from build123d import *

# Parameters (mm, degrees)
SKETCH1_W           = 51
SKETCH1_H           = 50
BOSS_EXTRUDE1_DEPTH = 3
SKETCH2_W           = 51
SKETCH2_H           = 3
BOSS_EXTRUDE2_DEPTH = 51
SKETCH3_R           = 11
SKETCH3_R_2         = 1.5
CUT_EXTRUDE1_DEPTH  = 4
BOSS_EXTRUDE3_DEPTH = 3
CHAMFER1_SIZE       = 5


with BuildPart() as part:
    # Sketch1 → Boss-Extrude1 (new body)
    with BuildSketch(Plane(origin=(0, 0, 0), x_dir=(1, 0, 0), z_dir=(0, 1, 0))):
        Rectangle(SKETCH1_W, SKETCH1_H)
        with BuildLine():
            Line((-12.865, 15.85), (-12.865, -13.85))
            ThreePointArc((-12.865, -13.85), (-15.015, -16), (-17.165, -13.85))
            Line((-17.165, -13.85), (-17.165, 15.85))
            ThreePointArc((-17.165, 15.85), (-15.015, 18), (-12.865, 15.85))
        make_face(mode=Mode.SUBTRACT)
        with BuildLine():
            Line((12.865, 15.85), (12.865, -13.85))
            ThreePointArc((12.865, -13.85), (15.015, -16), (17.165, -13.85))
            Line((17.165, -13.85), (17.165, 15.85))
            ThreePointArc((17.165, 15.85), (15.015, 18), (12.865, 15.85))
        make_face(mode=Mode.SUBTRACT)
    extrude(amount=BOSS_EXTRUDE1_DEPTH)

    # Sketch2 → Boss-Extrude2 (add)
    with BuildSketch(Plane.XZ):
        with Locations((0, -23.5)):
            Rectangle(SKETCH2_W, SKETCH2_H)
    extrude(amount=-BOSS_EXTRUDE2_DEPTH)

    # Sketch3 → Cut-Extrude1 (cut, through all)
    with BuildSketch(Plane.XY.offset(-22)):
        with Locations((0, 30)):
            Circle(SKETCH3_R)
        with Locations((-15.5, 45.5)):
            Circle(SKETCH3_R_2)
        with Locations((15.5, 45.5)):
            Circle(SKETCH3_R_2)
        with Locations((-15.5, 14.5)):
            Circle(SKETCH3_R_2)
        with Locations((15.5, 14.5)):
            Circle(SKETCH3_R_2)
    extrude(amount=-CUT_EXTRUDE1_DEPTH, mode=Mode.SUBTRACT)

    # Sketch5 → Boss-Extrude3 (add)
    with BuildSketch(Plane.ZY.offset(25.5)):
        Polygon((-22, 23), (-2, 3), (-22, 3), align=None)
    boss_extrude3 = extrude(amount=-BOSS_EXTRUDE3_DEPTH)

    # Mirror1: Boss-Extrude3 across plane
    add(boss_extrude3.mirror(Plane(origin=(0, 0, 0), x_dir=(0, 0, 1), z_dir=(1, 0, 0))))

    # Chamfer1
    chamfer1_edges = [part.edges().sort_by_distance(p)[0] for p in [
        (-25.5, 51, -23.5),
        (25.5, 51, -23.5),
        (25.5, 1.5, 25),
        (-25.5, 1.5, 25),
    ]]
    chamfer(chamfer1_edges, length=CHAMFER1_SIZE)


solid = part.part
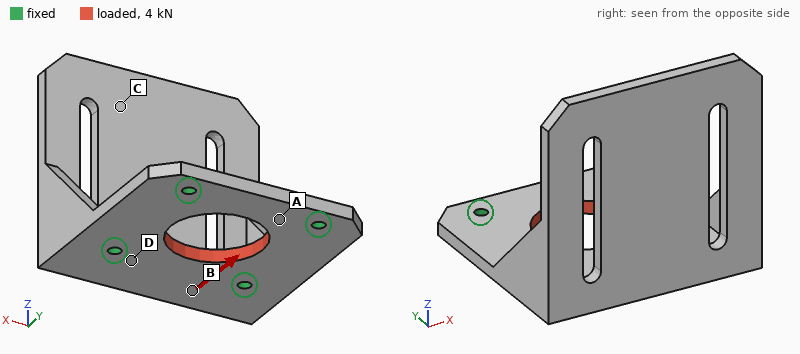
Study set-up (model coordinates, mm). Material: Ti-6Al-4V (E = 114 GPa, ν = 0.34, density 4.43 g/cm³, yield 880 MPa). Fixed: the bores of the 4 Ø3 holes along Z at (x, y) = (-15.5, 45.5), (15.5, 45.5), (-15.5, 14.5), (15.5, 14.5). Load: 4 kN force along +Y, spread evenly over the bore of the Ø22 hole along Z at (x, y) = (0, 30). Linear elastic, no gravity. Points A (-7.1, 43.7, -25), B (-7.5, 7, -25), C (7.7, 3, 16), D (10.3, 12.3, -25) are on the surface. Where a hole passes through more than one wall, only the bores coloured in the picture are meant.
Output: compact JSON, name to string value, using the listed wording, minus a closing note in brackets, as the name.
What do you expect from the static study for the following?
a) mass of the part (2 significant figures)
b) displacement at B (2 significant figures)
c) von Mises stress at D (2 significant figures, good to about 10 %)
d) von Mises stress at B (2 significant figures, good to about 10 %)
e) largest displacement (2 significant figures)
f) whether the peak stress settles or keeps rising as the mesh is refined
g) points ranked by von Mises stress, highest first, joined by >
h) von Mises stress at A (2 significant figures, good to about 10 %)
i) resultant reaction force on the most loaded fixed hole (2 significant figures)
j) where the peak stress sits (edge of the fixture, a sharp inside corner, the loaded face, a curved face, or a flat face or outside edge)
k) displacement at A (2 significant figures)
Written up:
{"mass of the part": "62 g", "displacement at B": "2.3 µm", "von Mises stress at D": "17 MPa", "von Mises stress at B": "13 MPa", "largest displacement": "7.6 µm", "whether the peak stress settles or keeps rising as the mesh is refined": "keeps rising", "points ranked by von Mises stress, highest first, joined by >": "A > D > B > C", "von Mises stress at A": "27 MPa", "resultant reaction force on the most loaded fixed hole": "1.0 kN", "where the peak stress sits": "edge of the fixture", "displacement at A": "4.9 µm"}
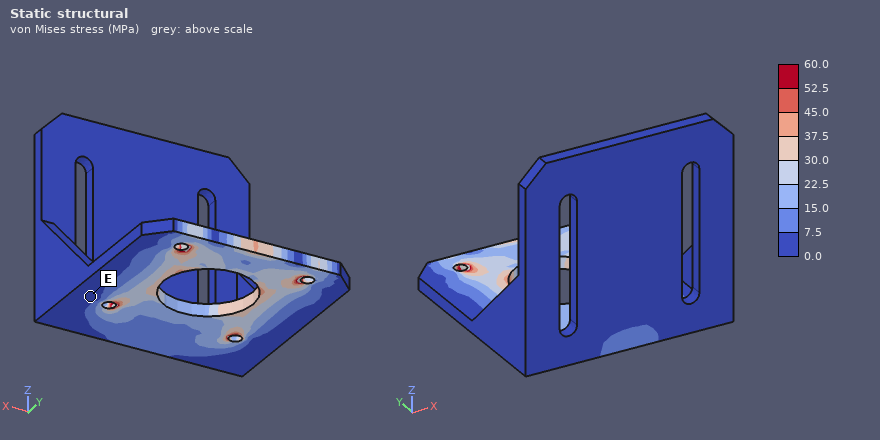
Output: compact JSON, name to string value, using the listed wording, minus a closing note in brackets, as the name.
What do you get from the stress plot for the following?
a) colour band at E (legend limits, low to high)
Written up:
{"colour band at E": "0.0 to 7.5 MPa"}
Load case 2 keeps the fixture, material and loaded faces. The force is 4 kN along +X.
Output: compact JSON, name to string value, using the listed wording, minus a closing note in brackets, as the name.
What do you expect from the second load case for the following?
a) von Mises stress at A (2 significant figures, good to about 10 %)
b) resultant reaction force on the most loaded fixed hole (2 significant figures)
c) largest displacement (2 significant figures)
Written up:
{"von Mises stress at A": "24 MPa", "resultant reaction force on the most loaded fixed hole": "1.0 kN", "largest displacement": "5.7 µm"}
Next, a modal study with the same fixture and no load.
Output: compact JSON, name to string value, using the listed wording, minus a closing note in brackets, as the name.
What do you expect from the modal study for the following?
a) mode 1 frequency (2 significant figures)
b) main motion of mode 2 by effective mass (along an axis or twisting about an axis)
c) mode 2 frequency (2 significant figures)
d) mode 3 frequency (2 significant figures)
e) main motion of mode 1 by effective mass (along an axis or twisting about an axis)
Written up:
{"mode 1 frequency": "1200 Hz", "main motion of mode 2 by effective mass": "along X", "mode 2 frequency": "2300 Hz", "mode 3 frequency": "4100 Hz", "main motion of mode 1 by effective mass": "along Y"}
